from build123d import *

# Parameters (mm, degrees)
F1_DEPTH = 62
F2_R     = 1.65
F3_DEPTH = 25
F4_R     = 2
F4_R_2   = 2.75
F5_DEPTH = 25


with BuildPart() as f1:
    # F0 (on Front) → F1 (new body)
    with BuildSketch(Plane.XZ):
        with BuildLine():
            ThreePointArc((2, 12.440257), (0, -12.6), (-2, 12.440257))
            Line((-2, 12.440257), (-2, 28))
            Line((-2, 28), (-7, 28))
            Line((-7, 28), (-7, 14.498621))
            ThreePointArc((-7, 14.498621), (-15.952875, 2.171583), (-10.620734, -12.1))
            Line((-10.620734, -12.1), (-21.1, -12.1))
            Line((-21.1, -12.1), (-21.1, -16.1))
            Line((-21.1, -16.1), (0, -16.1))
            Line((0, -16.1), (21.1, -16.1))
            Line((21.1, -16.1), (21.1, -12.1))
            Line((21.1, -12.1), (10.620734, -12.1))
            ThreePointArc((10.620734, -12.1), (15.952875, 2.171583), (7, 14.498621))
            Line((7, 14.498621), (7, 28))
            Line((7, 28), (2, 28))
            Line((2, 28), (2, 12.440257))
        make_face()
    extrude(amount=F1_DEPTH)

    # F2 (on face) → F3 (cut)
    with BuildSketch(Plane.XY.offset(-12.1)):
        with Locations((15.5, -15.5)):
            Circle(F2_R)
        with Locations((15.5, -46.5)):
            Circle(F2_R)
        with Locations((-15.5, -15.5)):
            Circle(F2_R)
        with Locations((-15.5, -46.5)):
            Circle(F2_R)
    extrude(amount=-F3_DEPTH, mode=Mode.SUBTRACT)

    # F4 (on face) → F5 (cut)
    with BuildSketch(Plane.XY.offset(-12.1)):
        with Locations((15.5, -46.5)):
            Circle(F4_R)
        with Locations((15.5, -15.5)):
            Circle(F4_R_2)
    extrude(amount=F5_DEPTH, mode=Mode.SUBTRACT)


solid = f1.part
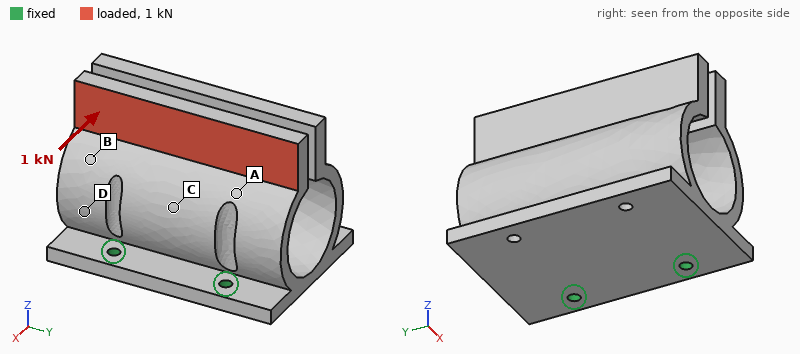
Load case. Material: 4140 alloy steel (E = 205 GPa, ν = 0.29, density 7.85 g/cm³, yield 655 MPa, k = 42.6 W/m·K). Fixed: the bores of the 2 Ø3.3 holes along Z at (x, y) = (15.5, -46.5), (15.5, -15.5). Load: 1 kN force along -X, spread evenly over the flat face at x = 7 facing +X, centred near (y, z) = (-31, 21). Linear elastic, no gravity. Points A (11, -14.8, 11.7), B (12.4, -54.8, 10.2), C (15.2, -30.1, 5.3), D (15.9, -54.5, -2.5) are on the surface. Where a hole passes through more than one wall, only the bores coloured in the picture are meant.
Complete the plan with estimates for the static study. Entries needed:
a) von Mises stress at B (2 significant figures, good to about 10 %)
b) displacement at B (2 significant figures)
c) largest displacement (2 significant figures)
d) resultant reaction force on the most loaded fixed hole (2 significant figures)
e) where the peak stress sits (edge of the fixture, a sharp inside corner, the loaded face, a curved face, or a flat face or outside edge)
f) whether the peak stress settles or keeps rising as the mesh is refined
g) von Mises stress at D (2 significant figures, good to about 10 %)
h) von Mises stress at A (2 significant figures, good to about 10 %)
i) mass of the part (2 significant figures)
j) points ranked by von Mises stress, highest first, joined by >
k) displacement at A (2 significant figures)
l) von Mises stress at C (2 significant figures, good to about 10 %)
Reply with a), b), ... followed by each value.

a) 87 MPa
b) 0.29 mm
c) 0.65 mm
d) 510 N
e) edge of the fixture
f) keeps rising
g) 170 MPa
h) 59 MPa
i) 260 g
j) D > C > B > A
k) 0.32 mm
l) 120 MPa
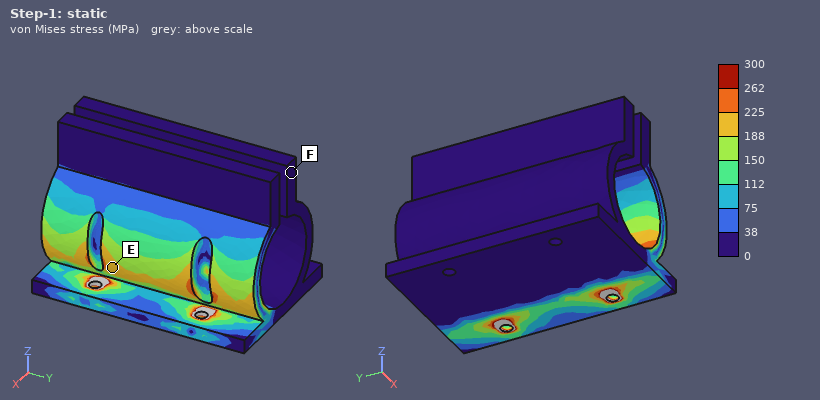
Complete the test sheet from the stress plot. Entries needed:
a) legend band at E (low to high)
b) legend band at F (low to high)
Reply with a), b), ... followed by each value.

a) 188 to 225 MPa
b) 0 to 38 MPa
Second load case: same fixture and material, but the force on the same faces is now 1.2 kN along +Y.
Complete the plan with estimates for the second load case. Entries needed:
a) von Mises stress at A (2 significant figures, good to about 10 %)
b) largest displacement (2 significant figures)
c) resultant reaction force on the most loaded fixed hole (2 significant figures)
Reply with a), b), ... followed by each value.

a) 19 MPa
b) 40 µm
c) 1.4 kN
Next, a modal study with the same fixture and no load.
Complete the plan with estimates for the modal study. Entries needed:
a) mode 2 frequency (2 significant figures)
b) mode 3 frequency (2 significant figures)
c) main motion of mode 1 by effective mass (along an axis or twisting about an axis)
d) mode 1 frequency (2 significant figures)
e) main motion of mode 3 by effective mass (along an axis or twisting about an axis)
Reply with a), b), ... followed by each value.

a) 1200 Hz
b) 1500 Hz
c) along X
d) 740 Hz
e) along Y
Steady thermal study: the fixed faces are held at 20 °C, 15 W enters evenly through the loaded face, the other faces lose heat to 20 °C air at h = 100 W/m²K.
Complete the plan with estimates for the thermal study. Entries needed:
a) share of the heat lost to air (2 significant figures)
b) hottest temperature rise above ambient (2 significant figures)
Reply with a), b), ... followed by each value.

a) 80 %
b) 34 K
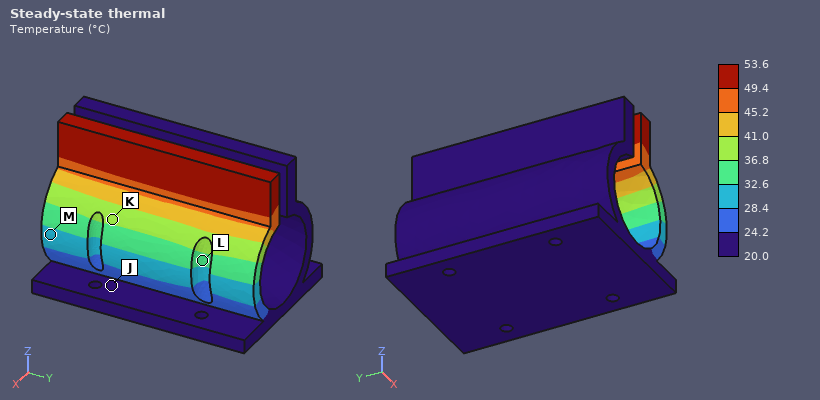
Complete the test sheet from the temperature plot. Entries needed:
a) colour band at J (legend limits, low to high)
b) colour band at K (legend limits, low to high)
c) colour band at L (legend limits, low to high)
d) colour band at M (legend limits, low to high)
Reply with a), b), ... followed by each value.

a) 20.0 to 24.2 °C
b) 36.8 to 41.0 °C
c) 32.6 to 36.8 °C
d) 28.4 to 32.6 °C
